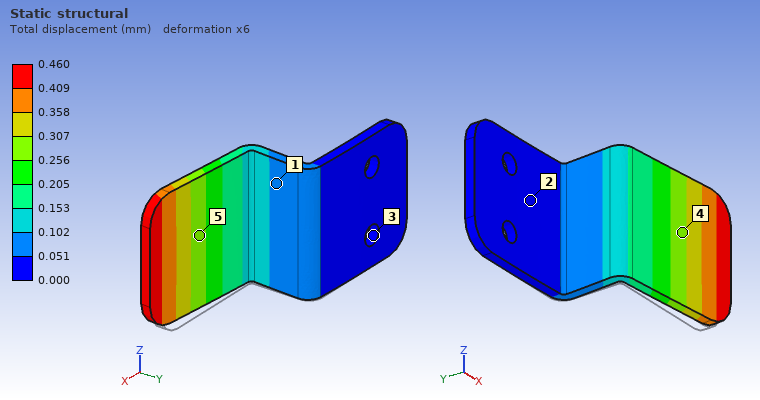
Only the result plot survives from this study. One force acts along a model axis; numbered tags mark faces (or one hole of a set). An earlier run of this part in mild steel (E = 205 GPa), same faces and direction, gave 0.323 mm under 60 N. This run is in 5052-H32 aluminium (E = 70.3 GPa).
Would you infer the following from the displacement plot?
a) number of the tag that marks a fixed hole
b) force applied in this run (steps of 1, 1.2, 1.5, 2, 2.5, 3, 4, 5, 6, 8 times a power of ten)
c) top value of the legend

3
30 N
0.460 mm
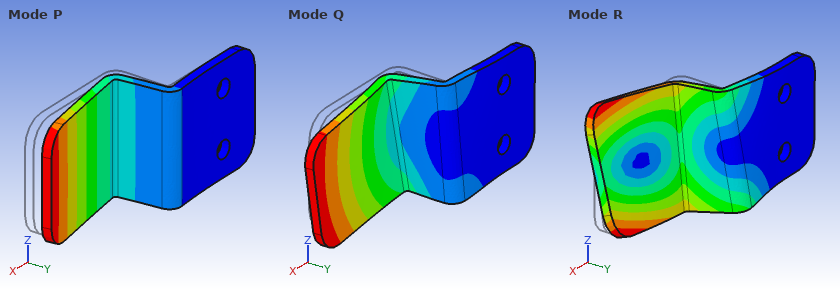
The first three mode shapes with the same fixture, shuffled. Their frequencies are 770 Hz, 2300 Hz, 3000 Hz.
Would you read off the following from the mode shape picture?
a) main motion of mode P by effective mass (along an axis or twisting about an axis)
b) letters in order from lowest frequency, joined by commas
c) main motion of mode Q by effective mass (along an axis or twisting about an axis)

along Y
P, Q, R
along Z
